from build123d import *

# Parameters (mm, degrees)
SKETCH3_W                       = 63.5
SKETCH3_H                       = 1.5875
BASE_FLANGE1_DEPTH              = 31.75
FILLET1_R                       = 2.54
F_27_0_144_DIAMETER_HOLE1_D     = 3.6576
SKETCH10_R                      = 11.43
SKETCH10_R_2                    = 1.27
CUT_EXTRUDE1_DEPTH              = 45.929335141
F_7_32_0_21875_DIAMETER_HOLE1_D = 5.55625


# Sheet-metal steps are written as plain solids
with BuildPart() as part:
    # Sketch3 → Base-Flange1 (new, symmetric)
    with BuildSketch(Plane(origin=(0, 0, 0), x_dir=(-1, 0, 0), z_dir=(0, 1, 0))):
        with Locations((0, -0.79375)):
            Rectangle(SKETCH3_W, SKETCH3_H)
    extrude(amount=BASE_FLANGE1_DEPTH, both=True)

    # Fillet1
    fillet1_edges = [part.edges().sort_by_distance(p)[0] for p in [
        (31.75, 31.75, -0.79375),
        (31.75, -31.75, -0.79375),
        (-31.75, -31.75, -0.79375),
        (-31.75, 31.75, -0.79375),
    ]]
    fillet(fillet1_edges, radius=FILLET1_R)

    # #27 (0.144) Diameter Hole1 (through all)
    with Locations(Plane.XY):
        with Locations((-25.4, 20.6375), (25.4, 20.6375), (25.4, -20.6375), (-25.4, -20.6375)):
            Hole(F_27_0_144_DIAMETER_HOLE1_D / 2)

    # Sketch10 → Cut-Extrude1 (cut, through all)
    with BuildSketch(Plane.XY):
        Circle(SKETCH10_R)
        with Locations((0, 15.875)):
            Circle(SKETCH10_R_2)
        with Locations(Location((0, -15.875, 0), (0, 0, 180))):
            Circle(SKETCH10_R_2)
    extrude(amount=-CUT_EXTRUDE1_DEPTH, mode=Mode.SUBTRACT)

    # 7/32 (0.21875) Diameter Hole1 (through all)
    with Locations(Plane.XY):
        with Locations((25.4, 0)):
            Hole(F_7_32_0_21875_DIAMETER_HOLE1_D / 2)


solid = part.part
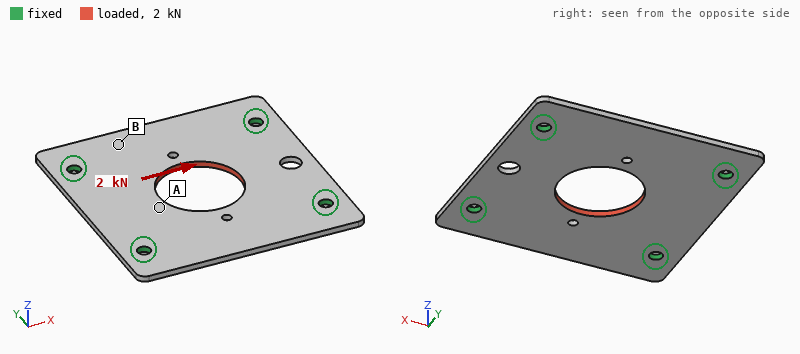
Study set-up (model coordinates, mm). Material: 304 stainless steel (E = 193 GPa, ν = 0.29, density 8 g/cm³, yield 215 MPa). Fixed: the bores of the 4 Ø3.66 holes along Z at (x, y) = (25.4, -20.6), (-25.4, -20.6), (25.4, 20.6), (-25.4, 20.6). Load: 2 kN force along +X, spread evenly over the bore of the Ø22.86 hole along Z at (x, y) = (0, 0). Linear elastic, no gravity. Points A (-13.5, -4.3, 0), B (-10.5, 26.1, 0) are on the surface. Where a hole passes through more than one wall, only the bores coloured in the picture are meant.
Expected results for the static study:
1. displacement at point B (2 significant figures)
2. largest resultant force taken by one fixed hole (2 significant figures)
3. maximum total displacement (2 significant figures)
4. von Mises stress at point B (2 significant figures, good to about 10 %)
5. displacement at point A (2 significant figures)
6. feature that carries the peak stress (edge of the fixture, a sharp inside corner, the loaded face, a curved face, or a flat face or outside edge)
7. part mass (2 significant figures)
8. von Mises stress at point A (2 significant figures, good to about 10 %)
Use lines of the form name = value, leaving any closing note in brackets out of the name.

displacement at point B = 0.93 µm
largest resultant force taken by one fixed hole = 530 N
maximum total displacement = 3.6 µm
von Mises stress at point B = 5.9 MPa
displacement at point A = 3.1 µm
feature that carries the peak stress = edge of the fixture
part mass = 45 g
von Mises stress at point A = 15 MPa
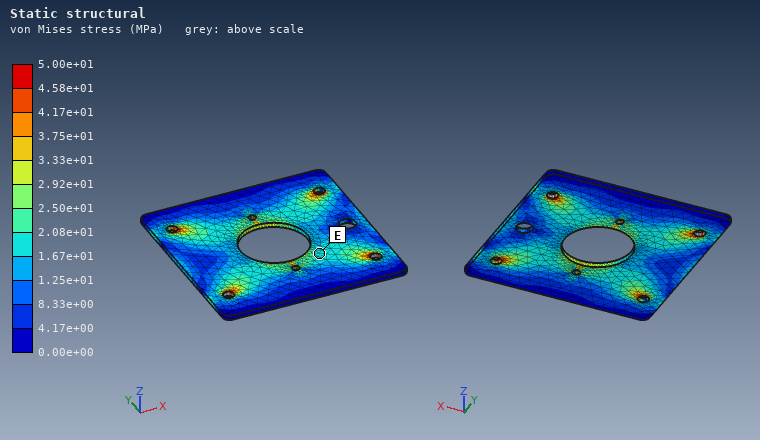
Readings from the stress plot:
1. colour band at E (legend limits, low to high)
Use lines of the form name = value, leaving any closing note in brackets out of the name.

colour band at E = 1.67e+01 to 2.08e+01 MPa
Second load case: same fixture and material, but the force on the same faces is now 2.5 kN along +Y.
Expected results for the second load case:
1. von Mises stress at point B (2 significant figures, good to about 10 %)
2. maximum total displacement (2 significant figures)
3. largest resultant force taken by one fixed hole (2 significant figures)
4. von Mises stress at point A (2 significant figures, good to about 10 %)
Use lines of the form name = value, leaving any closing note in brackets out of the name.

von Mises stress at point B = 14 MPa
maximum total displacement = 5.9 µm
largest resultant force taken by one fixed hole = 670 N
von Mises stress at point A = 35 MPa
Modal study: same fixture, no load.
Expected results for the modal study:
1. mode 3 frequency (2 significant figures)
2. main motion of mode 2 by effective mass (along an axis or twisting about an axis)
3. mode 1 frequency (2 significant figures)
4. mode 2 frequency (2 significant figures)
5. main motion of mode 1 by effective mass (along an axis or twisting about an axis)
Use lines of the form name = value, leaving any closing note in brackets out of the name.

mode 3 frequency = 3900 Hz
main motion of mode 2 by effective mass = twisting about X
mode 1 frequency = 2900 Hz
mode 2 frequency = 3300 Hz
main motion of mode 1 by effective mass = along Z
